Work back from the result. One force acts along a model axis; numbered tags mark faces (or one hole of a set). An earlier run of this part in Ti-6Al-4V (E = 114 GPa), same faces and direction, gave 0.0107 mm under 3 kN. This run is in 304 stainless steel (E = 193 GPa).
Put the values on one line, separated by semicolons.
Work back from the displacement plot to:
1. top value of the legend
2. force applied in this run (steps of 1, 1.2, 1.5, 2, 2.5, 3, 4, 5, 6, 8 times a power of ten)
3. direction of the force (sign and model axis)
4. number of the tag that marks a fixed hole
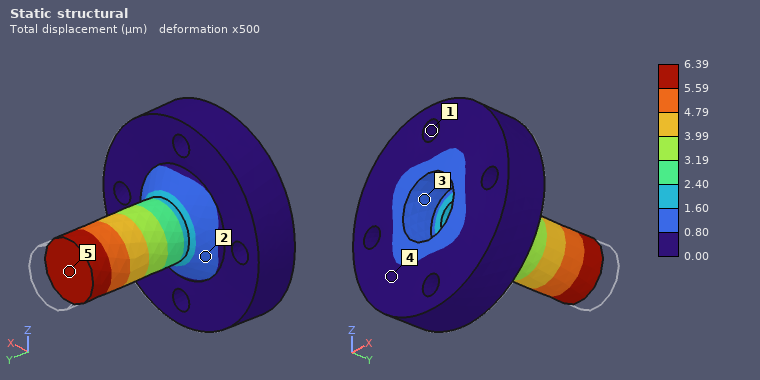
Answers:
6.39 µm; 3 kN; -Y; 1
